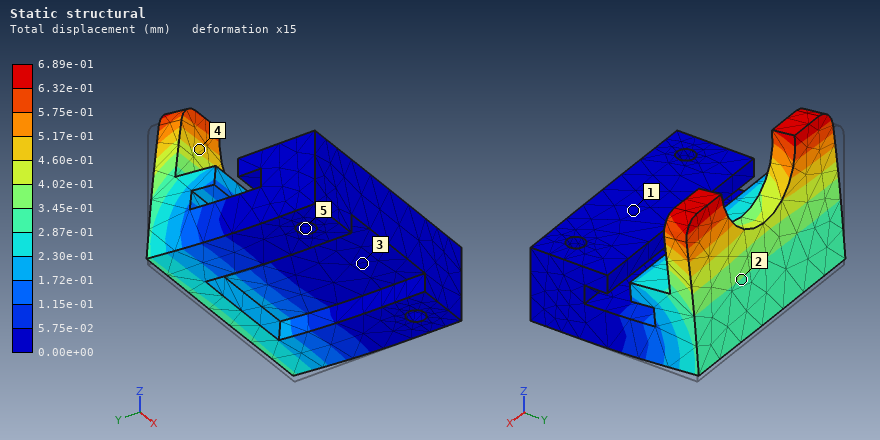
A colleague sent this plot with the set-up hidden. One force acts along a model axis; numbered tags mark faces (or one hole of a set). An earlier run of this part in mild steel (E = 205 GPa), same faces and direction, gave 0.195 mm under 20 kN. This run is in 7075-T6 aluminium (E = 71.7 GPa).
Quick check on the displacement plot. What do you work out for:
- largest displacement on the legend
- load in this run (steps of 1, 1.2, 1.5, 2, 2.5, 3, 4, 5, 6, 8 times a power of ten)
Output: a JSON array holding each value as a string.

["6.89e-01 mm", "25 kN"]
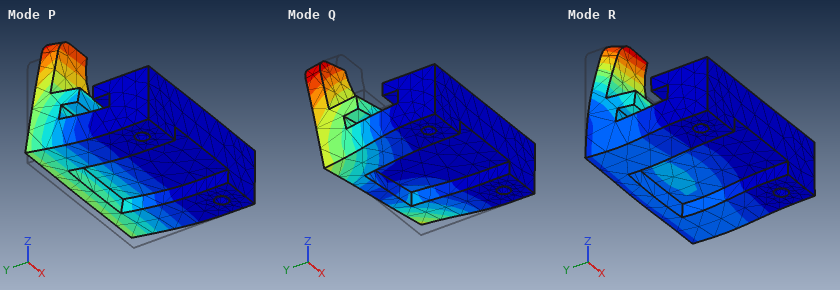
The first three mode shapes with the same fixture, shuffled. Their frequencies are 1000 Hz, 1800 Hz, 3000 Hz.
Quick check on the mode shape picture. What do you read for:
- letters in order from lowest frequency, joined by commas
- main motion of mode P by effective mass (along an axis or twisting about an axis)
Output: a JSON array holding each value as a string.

["P, Q, R", "along Z"]
